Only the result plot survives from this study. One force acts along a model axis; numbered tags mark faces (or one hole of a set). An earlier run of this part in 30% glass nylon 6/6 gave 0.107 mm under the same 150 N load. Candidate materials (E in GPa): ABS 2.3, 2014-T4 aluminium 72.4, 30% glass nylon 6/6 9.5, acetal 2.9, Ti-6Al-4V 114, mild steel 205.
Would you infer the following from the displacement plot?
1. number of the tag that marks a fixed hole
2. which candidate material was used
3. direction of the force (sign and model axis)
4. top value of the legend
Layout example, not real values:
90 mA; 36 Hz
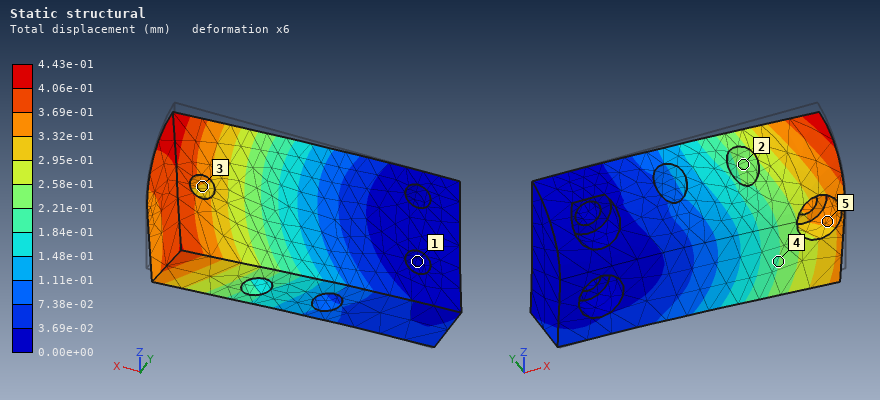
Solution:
1; ABS; -Z; 4.43e-01 mm
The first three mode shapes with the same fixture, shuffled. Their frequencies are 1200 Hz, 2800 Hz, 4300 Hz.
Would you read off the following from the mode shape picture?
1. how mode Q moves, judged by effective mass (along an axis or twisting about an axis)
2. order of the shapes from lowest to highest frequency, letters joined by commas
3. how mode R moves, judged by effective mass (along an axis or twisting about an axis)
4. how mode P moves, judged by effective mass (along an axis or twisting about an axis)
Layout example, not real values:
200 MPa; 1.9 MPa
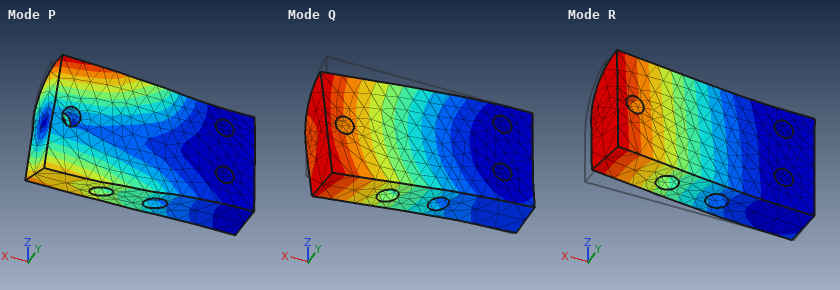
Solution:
along Z; R, Q, P; along Y; twisting about X
